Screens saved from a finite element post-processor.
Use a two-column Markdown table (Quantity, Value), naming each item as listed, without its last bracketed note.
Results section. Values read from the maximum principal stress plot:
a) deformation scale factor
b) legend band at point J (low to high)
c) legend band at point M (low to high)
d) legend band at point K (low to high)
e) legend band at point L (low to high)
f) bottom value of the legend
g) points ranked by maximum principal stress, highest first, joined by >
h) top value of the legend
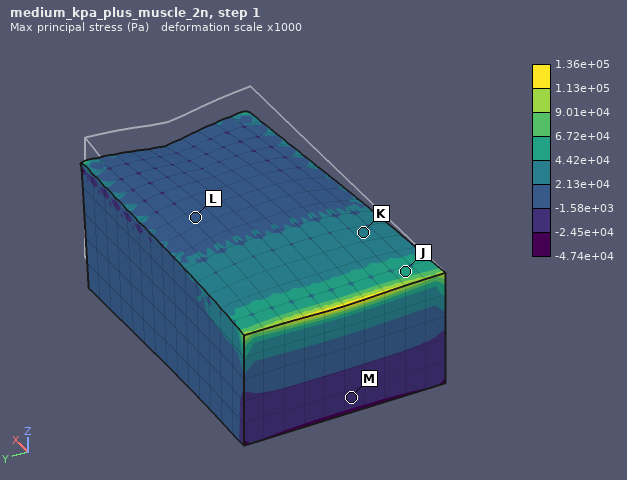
| Quantity | Value |
|---|---|
| deformation scale factor | 1000 |
| legend band at point J | 4.42e+04 to 6.72e+04 Pa |
| legend band at point M | -2.45e+04 to -1.58e+03 Pa |
| legend band at point K | 2.13e+04 to 4.42e+04 Pa |
| legend band at point L | -1.58e+03 to 2.13e+04 Pa |
| bottom value of the legend | -4.74e+04 Pa |
| points ranked by maximum principal stress, highest first, joined by > | J > K > L > M |
| top value of the legend | 1.36e+05 Pa |
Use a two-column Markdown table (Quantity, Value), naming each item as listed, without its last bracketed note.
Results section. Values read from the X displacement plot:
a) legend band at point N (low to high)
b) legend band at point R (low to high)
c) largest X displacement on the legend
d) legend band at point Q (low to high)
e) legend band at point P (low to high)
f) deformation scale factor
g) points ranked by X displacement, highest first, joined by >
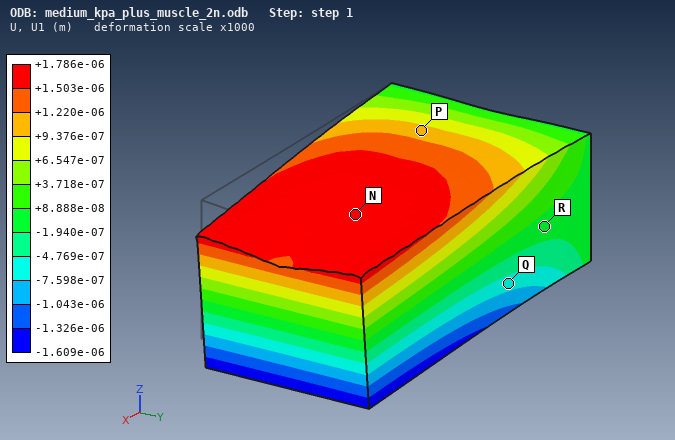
| Quantity | Value |
|---|---|
| legend band at point N | +1.503e-06 to +1.786e-06 m |
| legend band at point R | -1.940e-07 to +8.888e-08 m |
| largest X displacement on the legend | +1.786e-06 m |
| legend band at point Q | -7.598e-07 to -4.769e-07 m |
| legend band at point P | +9.376e-07 to +1.220e-06 m |
| deformation scale factor | 1000 |
| points ranked by X displacement, highest first, joined by > | N > P > R > Q |
